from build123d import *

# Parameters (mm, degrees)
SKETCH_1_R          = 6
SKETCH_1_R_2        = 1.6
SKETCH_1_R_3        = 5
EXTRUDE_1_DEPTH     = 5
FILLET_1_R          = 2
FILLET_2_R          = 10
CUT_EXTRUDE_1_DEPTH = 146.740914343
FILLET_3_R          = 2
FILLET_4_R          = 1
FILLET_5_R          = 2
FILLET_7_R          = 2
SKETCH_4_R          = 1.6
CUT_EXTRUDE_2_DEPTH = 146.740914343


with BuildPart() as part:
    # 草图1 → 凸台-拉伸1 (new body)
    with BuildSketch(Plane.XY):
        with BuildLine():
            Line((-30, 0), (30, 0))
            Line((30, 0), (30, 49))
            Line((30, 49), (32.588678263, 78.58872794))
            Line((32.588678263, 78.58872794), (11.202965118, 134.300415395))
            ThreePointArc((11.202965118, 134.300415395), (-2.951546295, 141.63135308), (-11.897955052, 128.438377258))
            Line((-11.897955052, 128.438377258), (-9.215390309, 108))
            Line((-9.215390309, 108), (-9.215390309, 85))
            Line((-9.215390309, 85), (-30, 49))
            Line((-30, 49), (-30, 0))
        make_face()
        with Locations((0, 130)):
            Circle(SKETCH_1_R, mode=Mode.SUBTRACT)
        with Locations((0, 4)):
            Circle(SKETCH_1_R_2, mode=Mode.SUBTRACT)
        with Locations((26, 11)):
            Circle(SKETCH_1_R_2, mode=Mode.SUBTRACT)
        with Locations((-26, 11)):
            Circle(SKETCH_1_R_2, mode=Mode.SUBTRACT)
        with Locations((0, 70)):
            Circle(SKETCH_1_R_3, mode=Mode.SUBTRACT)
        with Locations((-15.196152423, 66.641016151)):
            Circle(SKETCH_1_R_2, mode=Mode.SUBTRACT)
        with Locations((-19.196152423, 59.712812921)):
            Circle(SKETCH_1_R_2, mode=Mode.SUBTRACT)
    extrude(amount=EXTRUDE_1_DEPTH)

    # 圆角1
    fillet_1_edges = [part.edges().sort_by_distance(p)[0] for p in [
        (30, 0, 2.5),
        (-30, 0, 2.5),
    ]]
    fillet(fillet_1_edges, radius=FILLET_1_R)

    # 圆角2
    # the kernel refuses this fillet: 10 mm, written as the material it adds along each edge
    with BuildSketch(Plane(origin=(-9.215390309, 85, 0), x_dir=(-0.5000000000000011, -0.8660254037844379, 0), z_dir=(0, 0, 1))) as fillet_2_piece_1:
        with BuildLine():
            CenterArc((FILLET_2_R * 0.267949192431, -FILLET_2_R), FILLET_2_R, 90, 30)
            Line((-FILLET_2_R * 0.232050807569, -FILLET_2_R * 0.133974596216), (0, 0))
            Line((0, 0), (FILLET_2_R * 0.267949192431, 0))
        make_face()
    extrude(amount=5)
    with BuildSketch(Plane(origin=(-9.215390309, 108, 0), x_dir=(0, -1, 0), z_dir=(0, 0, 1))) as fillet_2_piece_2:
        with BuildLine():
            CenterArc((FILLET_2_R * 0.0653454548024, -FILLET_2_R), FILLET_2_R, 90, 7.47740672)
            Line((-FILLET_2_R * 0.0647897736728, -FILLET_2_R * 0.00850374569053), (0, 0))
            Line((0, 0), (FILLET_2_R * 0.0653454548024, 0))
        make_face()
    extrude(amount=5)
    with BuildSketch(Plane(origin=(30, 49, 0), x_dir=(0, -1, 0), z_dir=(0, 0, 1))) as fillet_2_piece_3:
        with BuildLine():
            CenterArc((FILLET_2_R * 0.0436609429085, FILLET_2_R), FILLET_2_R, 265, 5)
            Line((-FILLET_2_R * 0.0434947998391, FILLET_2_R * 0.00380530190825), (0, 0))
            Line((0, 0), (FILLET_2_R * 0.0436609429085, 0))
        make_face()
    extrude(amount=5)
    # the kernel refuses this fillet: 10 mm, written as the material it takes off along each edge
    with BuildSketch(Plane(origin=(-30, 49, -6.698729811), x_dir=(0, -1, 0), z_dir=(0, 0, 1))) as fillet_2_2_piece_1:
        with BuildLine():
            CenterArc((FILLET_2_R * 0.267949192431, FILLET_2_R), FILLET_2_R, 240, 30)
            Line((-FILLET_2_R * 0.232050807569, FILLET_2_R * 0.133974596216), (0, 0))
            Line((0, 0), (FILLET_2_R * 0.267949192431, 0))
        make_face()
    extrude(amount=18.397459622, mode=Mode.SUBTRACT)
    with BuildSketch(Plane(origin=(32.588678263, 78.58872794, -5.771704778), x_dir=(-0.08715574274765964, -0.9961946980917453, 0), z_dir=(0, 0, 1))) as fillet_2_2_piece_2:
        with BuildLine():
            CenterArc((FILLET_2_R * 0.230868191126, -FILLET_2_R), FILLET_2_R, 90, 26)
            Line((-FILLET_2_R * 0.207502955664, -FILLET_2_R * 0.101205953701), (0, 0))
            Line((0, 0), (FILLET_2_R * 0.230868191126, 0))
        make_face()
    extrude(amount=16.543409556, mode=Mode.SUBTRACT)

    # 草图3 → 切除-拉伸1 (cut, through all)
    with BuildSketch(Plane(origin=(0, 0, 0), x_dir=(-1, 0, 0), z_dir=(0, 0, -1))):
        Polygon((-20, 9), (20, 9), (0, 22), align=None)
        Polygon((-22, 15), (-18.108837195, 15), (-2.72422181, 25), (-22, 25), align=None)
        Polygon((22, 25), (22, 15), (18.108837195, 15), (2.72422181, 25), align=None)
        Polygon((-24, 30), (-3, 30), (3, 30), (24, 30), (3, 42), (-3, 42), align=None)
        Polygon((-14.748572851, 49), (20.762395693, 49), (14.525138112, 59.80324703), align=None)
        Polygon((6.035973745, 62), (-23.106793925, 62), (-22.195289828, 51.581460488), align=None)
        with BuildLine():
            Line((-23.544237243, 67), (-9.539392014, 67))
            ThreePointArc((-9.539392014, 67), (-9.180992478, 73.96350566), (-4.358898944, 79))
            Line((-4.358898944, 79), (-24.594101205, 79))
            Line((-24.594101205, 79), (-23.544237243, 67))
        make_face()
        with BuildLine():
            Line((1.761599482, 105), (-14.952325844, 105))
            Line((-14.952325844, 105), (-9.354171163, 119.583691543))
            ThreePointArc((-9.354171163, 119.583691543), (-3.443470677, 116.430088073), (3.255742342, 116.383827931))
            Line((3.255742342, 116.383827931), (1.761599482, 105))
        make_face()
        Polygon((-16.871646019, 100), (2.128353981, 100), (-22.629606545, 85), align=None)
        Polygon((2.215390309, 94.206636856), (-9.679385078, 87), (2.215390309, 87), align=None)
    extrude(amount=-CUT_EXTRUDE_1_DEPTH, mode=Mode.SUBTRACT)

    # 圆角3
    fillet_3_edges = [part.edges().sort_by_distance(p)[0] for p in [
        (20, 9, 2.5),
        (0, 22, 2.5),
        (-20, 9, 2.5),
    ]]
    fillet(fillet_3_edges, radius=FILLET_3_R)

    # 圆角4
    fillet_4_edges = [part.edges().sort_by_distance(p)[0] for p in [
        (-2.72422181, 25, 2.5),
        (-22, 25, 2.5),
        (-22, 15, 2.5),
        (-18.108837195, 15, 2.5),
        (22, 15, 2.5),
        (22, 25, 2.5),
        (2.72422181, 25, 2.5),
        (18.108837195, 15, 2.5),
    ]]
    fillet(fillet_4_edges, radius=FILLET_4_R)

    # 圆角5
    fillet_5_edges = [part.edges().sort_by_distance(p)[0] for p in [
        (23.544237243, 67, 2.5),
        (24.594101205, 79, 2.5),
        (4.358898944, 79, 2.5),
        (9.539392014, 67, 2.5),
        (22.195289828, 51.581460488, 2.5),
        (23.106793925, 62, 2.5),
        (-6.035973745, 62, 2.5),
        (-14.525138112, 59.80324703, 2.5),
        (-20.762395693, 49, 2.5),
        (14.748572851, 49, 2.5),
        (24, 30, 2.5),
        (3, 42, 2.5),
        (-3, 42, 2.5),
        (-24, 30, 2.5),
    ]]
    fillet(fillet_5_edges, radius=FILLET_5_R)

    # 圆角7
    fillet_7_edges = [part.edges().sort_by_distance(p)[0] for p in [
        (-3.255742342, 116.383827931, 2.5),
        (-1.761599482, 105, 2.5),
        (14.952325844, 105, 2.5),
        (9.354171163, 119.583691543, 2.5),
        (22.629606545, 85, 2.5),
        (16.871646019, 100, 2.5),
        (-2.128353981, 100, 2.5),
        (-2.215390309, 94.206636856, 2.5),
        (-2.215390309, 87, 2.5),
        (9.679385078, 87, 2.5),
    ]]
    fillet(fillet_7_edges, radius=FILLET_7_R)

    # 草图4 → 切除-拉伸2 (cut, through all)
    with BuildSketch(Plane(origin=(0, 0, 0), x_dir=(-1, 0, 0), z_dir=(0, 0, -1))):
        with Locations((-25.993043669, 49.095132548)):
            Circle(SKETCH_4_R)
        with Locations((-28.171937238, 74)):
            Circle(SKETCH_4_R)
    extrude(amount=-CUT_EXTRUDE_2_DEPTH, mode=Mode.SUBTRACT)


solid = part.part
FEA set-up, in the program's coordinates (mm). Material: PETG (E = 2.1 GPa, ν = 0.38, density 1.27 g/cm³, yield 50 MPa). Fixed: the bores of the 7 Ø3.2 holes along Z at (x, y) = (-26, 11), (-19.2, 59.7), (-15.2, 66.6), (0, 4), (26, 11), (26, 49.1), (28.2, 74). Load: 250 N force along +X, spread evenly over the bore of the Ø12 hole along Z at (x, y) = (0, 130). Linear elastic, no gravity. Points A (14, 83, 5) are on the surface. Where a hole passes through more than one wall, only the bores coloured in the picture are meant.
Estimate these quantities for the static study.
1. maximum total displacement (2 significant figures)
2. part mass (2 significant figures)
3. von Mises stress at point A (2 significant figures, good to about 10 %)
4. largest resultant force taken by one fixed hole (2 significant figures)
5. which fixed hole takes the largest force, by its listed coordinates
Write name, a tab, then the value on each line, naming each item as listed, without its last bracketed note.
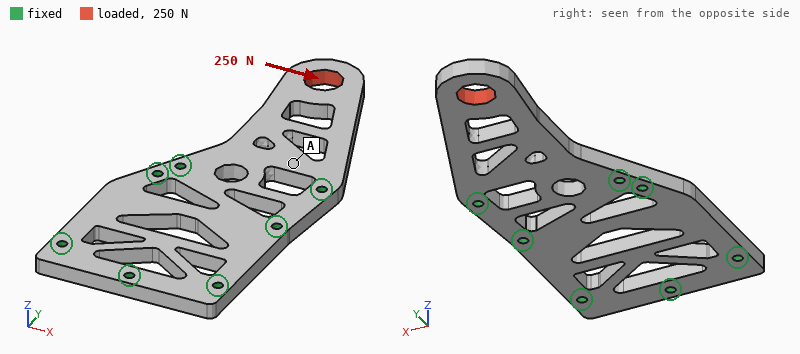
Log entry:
maximum total displacement	0.99 mm
part mass	29 g
von Mises stress at point A	2.4 MPa
largest resultant force taken by one fixed hole	370 N
which fixed hole takes the largest force, by its listed coordinates	(28.2, 74)
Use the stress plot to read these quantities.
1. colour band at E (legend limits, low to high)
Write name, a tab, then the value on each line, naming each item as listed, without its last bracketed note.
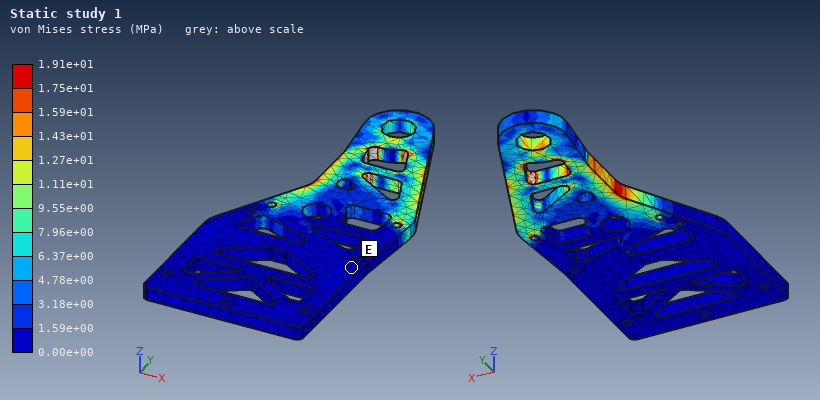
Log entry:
colour band at E	0.00e+00 to 1.59e+00 MPa
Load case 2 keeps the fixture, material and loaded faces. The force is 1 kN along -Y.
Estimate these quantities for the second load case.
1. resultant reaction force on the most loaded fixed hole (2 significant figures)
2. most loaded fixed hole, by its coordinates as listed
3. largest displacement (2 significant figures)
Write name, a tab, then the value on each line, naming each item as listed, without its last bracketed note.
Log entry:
resultant reaction force on the most loaded fixed hole	610 N
most loaded fixed hole, by its coordinates as listed	(-15.2, 66.6)
largest displacement	1.00 mm
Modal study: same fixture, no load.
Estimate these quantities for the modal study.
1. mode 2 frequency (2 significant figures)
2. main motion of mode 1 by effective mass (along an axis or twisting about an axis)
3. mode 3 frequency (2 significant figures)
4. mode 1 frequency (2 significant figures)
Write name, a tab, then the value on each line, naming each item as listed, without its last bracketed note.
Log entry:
mode 2 frequency	1000 Hz
main motion of mode 1 by effective mass	along Z
mode 3 frequency	1100 Hz
mode 1 frequency	220 Hz
